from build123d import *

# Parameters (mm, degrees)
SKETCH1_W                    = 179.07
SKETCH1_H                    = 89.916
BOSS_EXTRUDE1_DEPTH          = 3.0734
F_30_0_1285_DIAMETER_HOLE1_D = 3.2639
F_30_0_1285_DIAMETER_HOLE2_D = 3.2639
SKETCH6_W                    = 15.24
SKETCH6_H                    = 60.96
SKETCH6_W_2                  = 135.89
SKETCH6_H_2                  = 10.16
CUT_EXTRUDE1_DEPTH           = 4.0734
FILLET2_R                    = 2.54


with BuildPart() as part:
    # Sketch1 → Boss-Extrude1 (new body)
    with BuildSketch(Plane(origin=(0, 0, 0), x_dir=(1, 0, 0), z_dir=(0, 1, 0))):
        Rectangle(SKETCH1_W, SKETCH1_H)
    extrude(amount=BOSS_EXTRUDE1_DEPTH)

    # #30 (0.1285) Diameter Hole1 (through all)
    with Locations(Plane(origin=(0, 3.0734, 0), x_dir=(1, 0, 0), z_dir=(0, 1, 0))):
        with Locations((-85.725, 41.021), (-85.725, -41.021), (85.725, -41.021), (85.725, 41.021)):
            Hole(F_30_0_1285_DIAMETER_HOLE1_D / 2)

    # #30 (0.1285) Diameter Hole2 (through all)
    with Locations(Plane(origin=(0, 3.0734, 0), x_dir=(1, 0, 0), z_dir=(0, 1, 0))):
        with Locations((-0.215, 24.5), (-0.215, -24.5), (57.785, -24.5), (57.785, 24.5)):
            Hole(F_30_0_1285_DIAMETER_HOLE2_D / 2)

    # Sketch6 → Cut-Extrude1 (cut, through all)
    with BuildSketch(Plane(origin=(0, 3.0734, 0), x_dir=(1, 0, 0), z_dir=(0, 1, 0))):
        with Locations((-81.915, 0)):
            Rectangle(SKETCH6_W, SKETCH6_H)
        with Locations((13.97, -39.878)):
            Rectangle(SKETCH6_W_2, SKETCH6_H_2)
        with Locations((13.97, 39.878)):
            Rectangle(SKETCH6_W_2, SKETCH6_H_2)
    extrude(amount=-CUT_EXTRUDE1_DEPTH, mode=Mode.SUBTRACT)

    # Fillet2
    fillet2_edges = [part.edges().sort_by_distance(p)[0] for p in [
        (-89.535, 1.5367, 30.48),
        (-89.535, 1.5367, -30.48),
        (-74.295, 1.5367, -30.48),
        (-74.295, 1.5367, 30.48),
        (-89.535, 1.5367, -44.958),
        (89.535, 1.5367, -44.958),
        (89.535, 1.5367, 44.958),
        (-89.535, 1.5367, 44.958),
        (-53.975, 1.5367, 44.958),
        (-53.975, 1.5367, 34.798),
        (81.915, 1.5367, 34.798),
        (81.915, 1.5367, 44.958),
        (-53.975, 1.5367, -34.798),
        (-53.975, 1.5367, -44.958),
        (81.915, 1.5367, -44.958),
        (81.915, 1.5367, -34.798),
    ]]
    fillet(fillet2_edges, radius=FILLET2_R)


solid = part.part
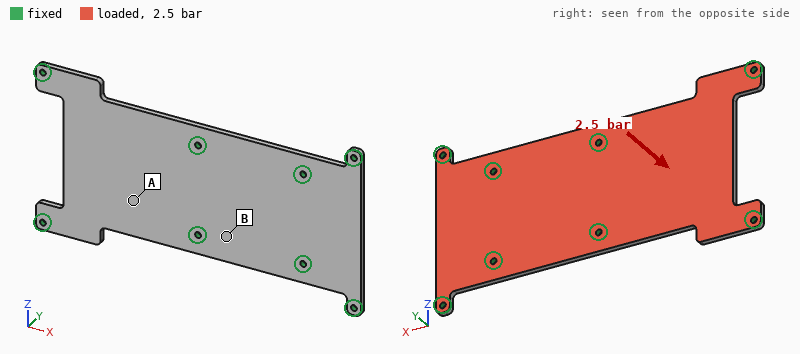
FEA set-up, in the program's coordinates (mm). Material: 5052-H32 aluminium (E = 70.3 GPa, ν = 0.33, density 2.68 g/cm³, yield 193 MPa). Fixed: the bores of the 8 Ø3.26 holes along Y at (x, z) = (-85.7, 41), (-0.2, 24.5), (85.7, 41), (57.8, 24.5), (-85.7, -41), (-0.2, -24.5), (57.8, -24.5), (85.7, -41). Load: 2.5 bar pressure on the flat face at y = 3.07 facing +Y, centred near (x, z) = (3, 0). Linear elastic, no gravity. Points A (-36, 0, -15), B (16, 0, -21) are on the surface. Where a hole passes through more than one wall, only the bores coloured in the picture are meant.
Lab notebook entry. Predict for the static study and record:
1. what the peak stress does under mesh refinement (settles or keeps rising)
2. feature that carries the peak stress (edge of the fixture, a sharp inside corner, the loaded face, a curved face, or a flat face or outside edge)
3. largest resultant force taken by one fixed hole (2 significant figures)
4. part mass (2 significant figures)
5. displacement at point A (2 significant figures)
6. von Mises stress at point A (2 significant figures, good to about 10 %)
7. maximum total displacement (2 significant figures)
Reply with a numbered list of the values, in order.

1. keeps rising
2. edge of the fixture
3. 680 N
4. 100 g
5. 0.33 mm
6. 43 MPa
7. 0.42 mm
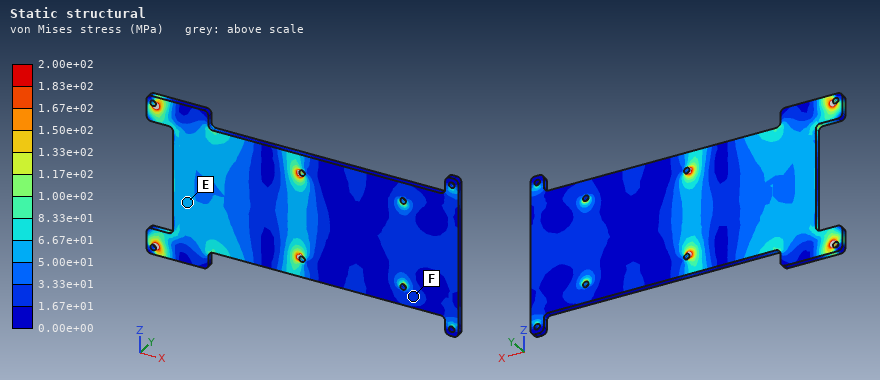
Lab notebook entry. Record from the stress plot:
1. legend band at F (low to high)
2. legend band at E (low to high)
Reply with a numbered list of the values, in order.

1. 1.67e+01 to 3.33e+01 MPa
2. 5.00e+01 to 6.67e+01 MPa
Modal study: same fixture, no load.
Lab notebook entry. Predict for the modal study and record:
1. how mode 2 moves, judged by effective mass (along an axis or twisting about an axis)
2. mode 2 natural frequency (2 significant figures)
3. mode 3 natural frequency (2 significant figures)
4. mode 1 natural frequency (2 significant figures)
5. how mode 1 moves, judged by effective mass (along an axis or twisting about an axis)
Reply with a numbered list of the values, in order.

1. twisting about X
2. 2600 Hz
3. 3300 Hz
4. 1500 Hz
5. along Y
